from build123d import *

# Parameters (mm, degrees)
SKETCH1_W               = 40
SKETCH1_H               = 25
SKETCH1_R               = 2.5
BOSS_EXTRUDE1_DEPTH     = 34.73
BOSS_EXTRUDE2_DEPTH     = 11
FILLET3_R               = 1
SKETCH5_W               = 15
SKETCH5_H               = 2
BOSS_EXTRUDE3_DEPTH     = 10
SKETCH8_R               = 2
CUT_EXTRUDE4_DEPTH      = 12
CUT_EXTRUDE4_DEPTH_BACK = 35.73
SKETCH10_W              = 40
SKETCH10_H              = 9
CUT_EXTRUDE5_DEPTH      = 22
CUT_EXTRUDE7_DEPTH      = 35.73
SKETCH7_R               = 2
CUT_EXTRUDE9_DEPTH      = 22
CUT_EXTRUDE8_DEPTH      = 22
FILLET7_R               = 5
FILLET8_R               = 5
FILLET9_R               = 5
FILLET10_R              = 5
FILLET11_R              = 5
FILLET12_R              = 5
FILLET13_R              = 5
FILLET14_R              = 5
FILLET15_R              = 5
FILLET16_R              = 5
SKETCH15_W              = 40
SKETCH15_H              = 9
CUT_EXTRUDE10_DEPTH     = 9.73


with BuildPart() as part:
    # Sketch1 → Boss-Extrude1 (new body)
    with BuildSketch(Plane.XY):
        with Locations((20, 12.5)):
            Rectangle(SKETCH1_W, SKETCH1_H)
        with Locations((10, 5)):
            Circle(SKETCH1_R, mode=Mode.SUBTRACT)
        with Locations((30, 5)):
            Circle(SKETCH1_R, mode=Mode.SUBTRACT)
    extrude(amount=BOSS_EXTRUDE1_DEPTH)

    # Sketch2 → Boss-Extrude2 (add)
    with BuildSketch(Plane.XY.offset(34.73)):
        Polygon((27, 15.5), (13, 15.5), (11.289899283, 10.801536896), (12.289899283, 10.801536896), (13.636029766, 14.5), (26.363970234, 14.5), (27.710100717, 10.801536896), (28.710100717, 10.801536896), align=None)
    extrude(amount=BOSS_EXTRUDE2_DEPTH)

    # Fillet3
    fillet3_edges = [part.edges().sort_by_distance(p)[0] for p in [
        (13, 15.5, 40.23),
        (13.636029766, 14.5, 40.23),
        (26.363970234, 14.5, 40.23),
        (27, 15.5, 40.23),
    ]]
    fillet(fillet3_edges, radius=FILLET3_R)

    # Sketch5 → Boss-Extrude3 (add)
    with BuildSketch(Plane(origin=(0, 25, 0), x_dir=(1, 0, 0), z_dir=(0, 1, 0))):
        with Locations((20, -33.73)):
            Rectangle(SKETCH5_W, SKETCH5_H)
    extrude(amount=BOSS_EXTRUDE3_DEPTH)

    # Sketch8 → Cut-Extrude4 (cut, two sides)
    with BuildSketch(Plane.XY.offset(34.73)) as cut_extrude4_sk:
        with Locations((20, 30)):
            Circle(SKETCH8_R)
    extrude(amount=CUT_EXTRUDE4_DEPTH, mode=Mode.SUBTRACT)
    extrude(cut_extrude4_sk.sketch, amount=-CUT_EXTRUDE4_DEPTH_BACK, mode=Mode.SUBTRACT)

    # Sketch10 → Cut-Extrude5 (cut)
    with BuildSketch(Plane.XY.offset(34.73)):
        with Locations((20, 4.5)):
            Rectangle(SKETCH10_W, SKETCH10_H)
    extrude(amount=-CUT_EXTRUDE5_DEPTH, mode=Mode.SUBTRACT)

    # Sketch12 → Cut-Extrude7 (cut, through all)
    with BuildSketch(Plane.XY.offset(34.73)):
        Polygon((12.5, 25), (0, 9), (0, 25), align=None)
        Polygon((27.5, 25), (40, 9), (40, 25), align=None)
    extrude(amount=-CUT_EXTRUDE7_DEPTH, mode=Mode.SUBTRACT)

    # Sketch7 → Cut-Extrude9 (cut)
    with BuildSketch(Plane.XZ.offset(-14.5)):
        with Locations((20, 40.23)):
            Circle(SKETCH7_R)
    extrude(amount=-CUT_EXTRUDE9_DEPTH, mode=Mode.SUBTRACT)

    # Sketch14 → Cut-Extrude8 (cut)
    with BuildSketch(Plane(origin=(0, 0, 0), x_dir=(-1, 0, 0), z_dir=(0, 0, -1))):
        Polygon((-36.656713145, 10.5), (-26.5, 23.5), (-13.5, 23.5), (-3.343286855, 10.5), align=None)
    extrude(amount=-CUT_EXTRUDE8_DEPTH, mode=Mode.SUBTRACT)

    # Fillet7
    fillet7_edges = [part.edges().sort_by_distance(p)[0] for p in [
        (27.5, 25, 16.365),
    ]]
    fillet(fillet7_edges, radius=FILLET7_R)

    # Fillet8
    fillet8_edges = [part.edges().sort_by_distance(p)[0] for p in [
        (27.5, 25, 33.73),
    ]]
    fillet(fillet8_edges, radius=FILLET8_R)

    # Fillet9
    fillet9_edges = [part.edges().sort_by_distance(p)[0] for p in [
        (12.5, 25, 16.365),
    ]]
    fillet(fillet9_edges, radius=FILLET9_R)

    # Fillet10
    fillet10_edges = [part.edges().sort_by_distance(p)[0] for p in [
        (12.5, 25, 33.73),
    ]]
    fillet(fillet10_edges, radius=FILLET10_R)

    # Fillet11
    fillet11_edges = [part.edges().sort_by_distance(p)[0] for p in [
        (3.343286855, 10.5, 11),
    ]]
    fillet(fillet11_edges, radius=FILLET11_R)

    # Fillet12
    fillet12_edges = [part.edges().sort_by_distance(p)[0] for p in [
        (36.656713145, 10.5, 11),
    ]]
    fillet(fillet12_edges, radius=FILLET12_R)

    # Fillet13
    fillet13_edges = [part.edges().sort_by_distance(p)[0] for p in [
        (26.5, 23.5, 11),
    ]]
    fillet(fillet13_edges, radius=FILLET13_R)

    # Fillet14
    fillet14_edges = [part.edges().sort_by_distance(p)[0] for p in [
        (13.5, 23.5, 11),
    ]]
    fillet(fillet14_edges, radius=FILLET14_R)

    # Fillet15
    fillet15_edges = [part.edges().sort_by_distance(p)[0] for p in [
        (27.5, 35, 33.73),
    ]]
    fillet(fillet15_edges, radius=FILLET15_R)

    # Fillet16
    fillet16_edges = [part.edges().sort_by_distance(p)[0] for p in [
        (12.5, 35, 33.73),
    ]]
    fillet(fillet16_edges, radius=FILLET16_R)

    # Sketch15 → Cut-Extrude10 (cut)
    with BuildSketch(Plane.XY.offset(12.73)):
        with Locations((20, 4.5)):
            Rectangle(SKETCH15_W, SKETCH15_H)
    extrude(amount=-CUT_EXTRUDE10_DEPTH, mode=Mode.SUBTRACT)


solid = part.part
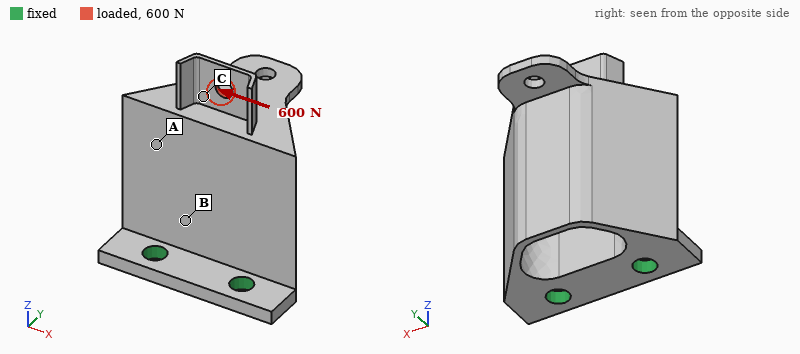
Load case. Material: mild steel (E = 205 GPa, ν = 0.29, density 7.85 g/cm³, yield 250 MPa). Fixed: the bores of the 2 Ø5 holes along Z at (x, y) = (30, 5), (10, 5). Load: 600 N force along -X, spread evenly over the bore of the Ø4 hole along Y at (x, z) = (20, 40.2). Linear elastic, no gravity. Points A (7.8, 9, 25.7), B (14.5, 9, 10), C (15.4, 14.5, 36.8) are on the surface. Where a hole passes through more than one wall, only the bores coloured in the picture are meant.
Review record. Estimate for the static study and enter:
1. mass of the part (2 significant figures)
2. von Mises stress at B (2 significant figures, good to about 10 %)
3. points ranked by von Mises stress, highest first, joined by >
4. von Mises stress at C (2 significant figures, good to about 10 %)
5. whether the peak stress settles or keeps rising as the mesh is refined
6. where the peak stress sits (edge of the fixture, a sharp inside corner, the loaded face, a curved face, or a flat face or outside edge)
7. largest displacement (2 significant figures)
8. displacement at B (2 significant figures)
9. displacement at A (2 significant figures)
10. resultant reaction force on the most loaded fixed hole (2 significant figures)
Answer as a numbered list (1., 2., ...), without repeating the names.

1. 87 g
2. 35 MPa
3. C > B > A
4. 80 MPa
5. keeps rising
6. edge of the fixture
7. 33 µm
8. 5.0 µm
9. 14 µm
10. 1.0 kN
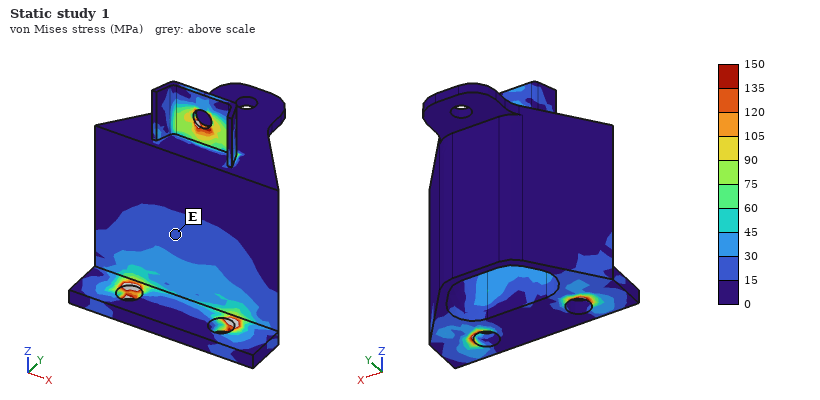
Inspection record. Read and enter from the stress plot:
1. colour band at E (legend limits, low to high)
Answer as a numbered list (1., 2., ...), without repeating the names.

1. 15 to 30 MPa
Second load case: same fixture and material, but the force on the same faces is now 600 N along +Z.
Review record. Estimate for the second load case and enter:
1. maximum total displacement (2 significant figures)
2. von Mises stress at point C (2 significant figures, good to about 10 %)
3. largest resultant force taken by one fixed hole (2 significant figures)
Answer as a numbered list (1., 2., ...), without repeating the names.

1. 69 µm
2. 40 MPa
3. 300 N
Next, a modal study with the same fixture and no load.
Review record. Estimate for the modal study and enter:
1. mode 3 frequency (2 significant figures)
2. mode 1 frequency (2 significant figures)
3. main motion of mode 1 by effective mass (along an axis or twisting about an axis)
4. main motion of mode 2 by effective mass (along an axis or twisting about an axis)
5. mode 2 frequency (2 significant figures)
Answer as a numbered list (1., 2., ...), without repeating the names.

1. 8200 Hz
2. 1200 Hz
3. along Y
4. along X
5. 4900 Hz
